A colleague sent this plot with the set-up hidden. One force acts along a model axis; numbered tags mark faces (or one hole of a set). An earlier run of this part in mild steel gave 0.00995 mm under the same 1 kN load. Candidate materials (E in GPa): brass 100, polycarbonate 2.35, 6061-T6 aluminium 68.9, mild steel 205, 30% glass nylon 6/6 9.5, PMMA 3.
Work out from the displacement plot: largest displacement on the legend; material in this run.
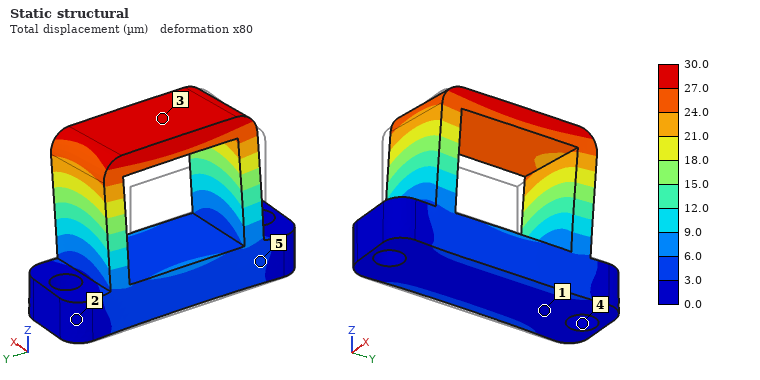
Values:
30.0 µm
6061-T6 aluminium
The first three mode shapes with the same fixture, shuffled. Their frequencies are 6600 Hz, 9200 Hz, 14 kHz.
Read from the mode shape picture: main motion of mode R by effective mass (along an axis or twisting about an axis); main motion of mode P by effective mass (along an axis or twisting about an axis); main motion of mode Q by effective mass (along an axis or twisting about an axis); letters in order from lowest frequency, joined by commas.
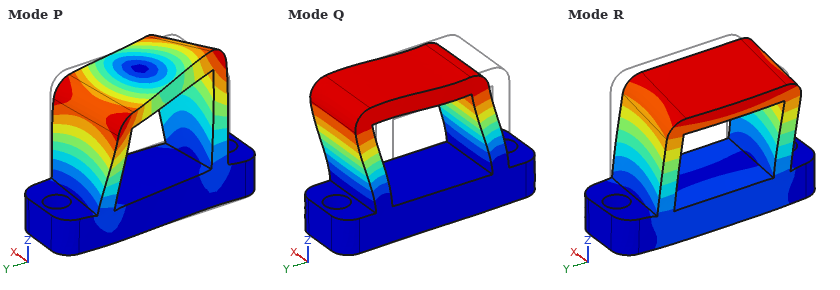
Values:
along X
twisting about Z
along Y
Q, R, P
